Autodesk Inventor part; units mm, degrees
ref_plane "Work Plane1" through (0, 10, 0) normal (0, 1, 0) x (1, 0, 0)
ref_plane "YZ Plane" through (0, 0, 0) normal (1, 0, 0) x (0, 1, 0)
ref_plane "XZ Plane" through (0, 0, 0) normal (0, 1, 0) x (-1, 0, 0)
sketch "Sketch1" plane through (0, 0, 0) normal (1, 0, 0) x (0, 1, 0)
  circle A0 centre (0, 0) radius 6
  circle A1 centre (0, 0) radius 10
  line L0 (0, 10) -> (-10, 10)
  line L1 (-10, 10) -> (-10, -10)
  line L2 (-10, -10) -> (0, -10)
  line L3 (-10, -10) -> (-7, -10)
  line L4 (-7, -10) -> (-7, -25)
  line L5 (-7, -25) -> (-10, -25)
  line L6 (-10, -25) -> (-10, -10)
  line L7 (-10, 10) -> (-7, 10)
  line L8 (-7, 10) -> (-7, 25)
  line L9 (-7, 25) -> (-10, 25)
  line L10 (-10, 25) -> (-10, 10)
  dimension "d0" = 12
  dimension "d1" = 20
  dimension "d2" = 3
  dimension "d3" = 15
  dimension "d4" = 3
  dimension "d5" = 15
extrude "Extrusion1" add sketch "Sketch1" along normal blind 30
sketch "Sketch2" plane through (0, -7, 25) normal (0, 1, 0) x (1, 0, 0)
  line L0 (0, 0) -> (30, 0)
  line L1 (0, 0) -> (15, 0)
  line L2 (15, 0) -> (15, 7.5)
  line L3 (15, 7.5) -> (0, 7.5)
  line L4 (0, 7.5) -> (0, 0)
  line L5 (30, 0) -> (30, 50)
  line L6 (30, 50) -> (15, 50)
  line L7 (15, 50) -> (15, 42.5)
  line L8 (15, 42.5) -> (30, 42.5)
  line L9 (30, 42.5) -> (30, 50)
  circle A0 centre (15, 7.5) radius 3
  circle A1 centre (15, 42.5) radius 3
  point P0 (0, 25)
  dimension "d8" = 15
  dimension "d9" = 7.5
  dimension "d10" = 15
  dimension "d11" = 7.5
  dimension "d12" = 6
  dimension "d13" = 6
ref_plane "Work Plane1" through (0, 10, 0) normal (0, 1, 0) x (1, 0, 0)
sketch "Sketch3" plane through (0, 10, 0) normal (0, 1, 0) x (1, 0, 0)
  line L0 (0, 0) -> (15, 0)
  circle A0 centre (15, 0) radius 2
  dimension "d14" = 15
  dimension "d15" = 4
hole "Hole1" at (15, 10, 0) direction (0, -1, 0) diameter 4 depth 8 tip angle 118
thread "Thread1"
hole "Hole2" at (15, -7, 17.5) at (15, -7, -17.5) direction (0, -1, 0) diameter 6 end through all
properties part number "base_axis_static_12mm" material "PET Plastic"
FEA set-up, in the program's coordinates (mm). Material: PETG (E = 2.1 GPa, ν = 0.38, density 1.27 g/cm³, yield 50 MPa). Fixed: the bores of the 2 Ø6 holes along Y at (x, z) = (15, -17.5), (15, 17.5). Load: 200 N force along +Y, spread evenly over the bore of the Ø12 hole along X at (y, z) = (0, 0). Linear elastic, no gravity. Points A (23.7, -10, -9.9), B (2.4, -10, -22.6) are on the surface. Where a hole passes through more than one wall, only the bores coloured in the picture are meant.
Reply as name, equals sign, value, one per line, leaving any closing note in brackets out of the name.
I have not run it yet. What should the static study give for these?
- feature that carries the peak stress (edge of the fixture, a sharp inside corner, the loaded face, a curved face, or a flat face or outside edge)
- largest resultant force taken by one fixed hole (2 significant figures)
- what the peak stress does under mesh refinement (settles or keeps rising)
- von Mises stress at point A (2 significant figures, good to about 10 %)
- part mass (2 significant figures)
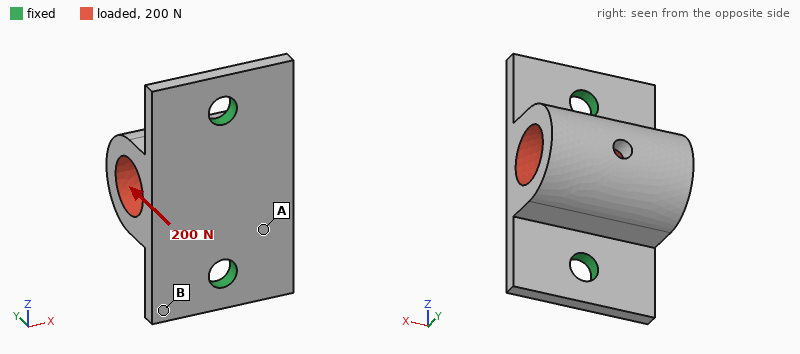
feature that carries the peak stress = edge of the fixture
largest resultant force taken by one fixed hole = 110 N
what the peak stress does under mesh refinement = keeps rising
von Mises stress at point A = 3.1 MPa
part mass = 12 g
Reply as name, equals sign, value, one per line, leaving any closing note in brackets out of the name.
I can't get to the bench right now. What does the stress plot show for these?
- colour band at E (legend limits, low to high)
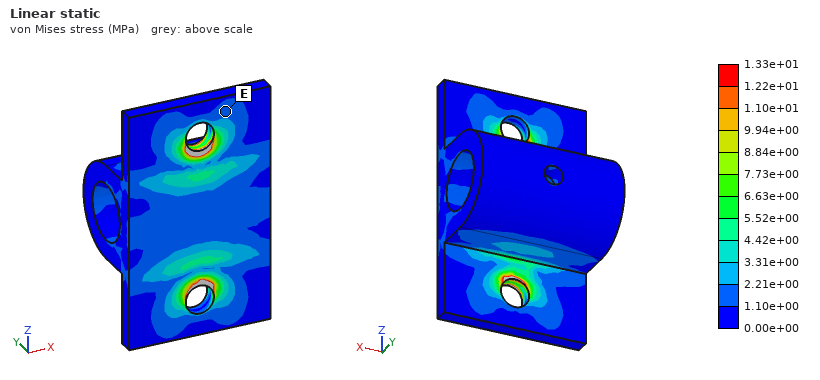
colour band at E = 1.10e+00 to 2.21e+00 MPa
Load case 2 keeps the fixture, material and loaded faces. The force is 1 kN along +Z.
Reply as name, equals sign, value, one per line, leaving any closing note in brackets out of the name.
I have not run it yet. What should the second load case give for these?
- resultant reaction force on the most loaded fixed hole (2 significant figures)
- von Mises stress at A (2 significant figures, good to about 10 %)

resultant reaction force on the most loaded fixed hole = 590 N
von Mises stress at A = 11 MPa
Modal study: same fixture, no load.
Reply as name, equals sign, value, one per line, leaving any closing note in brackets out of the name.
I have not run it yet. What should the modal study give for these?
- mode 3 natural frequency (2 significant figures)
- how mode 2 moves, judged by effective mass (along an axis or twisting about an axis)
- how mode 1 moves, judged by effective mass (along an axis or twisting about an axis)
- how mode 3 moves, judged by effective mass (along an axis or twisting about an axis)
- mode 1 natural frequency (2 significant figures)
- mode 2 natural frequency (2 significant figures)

mode 3 natural frequency = 3100 Hz
how mode 2 moves, judged by effective mass = along Y
how mode 1 moves, judged by effective mass = along X
how mode 3 moves, judged by effective mass = along Z
mode 1 natural frequency = 1200 Hz
mode 2 natural frequency = 2800 Hz
